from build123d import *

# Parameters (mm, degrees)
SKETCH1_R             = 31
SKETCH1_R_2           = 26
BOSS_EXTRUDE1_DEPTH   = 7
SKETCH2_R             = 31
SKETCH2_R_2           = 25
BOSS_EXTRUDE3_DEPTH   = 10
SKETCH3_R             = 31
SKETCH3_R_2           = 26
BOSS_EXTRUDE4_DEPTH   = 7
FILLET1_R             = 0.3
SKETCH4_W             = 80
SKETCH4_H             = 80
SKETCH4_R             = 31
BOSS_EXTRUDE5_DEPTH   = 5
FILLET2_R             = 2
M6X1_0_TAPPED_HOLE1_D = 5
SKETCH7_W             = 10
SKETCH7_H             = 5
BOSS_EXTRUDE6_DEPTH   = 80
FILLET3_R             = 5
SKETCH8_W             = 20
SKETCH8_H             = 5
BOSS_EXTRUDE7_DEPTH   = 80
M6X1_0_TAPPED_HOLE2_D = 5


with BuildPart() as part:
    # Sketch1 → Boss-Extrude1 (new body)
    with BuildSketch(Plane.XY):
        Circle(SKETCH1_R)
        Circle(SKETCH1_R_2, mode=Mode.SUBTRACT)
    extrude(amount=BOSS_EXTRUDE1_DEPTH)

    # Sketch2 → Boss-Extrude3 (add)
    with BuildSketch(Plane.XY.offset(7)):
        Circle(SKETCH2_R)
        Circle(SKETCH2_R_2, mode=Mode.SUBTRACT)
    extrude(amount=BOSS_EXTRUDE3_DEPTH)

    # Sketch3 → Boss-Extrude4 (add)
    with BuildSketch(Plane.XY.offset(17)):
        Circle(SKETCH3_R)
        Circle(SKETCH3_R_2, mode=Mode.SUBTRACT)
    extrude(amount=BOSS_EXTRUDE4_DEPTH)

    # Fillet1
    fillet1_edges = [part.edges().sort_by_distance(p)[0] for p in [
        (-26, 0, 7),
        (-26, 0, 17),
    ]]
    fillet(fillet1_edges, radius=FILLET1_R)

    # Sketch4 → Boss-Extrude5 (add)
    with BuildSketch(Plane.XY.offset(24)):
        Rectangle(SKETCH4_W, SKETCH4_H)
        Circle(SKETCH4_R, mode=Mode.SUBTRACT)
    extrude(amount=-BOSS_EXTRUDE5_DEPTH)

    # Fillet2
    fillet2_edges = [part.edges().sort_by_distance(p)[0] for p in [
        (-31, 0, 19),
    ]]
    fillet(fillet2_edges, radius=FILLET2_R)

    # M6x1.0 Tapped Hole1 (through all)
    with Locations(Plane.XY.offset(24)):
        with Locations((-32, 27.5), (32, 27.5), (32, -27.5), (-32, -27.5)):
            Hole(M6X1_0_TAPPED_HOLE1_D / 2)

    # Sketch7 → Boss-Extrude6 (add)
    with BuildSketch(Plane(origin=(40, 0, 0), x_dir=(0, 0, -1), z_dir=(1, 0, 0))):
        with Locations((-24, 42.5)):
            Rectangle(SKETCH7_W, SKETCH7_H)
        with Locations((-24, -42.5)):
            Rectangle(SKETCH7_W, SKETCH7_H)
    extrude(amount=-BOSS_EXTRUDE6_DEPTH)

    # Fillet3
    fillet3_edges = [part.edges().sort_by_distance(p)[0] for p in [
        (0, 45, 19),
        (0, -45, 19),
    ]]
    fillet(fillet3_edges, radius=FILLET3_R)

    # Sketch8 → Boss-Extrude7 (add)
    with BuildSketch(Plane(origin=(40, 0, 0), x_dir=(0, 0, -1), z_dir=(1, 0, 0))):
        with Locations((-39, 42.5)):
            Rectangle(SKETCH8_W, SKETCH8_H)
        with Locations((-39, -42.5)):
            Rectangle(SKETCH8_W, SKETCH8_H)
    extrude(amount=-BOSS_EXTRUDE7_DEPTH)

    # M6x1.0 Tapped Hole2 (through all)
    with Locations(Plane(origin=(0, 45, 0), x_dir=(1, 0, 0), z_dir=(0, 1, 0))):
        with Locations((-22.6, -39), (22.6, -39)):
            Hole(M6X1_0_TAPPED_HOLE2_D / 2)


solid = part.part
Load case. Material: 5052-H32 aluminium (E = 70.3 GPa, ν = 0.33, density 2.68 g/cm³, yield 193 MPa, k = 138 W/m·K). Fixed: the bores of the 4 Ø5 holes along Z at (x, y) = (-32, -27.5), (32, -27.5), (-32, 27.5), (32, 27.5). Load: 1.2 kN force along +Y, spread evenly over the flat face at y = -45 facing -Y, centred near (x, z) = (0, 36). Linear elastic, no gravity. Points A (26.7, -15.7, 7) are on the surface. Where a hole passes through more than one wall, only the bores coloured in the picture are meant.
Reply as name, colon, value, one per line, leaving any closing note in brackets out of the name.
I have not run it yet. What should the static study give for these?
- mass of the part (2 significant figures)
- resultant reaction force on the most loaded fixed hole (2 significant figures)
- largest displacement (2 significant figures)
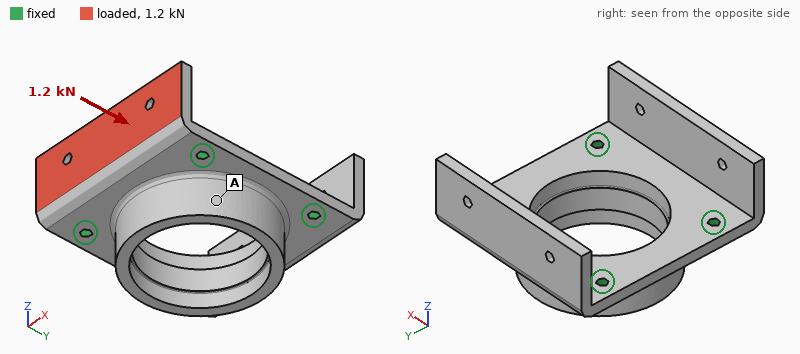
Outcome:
mass of the part: 170 g
resultant reaction force on the most loaded fixed hole: 630 N
largest displacement: 0.18 mm
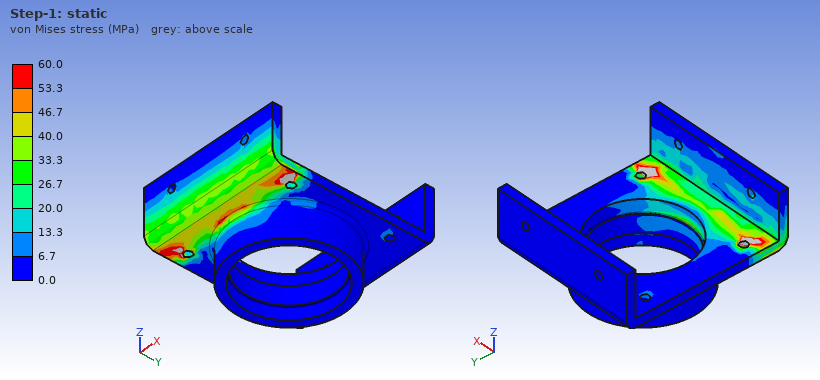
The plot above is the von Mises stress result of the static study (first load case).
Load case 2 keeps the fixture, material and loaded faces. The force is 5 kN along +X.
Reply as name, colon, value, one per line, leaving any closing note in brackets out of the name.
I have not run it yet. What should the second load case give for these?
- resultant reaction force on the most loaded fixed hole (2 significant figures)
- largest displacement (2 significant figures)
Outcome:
resultant reaction force on the most loaded fixed hole: 3.0 kN
largest displacement: 88 µm
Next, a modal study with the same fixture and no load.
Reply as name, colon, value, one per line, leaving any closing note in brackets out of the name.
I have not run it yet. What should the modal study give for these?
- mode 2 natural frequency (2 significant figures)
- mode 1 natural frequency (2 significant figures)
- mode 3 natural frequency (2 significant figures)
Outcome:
mode 2 natural frequency: 2900 Hz
mode 1 natural frequency: 2900 Hz
mode 3 natural frequency: 4600 Hz
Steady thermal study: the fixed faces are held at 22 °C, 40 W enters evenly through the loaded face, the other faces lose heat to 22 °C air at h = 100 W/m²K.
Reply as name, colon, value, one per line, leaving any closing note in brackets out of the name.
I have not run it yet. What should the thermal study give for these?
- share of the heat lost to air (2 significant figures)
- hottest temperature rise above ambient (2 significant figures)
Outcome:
share of the heat lost to air: 27 %
hottest temperature rise above ambient: 22 K
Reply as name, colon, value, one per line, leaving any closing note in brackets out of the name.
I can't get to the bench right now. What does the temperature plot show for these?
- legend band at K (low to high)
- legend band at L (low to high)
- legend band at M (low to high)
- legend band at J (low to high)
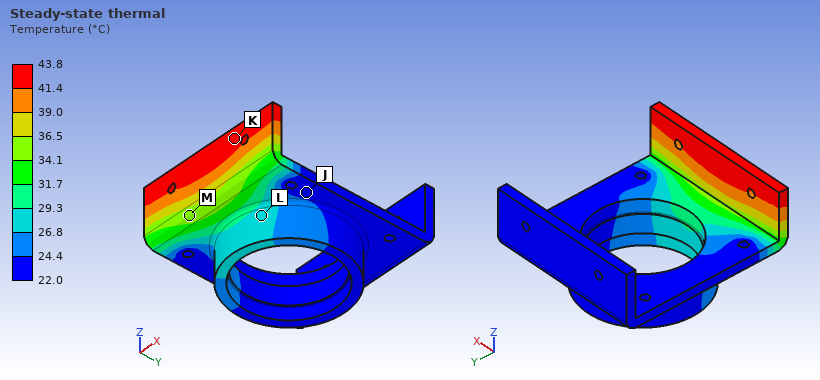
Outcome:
legend band at K: 41.4 to 43.8 °C
legend band at L: 26.8 to 29.3 °C
legend band at M: 34.1 to 36.5 °C
legend band at J: 22.0 to 24.4 °C
